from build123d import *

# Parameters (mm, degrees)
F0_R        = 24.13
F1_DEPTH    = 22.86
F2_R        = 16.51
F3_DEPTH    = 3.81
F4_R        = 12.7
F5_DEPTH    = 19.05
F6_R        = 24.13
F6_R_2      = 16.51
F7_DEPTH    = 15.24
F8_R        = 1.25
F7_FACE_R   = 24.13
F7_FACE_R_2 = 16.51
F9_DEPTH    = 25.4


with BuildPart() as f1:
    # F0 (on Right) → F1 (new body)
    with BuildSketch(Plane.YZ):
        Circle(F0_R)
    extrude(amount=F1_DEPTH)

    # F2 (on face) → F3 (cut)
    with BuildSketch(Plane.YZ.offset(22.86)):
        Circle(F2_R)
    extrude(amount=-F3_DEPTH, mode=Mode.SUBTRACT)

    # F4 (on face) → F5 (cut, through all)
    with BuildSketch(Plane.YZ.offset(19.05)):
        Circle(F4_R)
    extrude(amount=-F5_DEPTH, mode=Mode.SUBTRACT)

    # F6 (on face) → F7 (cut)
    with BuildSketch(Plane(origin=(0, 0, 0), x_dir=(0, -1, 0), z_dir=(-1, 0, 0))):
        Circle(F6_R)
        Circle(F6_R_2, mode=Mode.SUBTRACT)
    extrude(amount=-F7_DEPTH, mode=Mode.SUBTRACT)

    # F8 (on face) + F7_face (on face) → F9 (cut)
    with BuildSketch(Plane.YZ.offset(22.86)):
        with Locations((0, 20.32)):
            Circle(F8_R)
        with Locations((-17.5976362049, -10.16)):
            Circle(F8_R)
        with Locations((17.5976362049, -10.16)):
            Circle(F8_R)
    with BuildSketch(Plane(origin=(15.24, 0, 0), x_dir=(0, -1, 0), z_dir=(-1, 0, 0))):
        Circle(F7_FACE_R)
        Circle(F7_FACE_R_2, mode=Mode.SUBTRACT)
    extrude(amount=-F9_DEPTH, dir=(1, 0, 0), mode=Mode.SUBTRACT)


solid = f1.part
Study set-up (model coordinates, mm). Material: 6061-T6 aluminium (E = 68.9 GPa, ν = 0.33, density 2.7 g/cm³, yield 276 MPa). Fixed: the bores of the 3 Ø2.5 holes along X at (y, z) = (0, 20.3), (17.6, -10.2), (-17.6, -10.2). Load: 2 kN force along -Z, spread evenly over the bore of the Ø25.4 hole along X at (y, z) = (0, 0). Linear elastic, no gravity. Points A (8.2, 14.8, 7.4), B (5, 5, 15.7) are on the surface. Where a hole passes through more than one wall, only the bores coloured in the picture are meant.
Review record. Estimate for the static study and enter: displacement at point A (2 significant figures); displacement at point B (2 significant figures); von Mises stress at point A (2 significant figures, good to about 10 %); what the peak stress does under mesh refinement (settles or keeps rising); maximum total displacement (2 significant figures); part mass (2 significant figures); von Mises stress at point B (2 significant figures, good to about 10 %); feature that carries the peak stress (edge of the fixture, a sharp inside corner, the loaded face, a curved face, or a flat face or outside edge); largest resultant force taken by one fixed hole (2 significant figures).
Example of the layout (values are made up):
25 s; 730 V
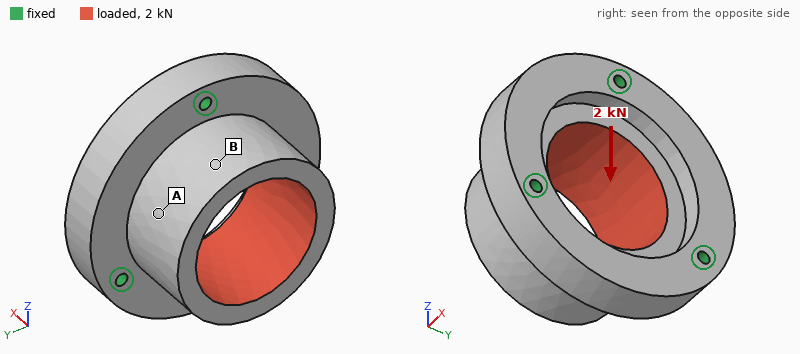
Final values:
6.1 µm; 5.3 µm; 9.7 MPa; keeps rising; 14 µm; 38 g; 2.8 MPa; edge of the fixture; 780 N
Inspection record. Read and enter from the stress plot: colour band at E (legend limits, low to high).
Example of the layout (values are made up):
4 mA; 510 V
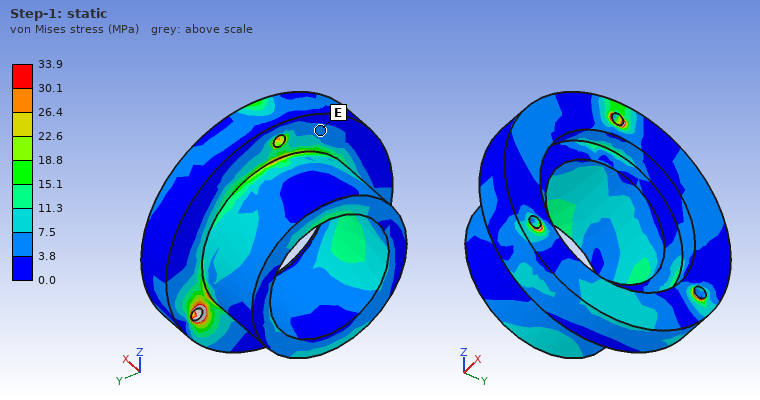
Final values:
3.8 to 7.5 MPa
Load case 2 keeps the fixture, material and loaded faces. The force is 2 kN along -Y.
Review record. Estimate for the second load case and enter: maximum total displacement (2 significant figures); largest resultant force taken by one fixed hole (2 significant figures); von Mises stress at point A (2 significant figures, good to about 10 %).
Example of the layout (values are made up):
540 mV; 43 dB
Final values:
12 µm; 780 N; 7.9 MPa
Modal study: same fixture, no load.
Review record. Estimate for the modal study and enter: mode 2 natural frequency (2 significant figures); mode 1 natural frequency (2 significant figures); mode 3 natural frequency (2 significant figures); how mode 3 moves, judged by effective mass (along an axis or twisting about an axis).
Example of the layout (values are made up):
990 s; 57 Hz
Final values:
13 kHz; 13 kHz; 19 kHz; along X
